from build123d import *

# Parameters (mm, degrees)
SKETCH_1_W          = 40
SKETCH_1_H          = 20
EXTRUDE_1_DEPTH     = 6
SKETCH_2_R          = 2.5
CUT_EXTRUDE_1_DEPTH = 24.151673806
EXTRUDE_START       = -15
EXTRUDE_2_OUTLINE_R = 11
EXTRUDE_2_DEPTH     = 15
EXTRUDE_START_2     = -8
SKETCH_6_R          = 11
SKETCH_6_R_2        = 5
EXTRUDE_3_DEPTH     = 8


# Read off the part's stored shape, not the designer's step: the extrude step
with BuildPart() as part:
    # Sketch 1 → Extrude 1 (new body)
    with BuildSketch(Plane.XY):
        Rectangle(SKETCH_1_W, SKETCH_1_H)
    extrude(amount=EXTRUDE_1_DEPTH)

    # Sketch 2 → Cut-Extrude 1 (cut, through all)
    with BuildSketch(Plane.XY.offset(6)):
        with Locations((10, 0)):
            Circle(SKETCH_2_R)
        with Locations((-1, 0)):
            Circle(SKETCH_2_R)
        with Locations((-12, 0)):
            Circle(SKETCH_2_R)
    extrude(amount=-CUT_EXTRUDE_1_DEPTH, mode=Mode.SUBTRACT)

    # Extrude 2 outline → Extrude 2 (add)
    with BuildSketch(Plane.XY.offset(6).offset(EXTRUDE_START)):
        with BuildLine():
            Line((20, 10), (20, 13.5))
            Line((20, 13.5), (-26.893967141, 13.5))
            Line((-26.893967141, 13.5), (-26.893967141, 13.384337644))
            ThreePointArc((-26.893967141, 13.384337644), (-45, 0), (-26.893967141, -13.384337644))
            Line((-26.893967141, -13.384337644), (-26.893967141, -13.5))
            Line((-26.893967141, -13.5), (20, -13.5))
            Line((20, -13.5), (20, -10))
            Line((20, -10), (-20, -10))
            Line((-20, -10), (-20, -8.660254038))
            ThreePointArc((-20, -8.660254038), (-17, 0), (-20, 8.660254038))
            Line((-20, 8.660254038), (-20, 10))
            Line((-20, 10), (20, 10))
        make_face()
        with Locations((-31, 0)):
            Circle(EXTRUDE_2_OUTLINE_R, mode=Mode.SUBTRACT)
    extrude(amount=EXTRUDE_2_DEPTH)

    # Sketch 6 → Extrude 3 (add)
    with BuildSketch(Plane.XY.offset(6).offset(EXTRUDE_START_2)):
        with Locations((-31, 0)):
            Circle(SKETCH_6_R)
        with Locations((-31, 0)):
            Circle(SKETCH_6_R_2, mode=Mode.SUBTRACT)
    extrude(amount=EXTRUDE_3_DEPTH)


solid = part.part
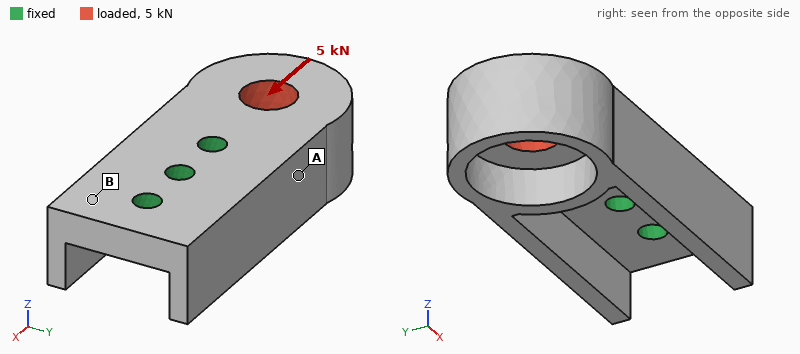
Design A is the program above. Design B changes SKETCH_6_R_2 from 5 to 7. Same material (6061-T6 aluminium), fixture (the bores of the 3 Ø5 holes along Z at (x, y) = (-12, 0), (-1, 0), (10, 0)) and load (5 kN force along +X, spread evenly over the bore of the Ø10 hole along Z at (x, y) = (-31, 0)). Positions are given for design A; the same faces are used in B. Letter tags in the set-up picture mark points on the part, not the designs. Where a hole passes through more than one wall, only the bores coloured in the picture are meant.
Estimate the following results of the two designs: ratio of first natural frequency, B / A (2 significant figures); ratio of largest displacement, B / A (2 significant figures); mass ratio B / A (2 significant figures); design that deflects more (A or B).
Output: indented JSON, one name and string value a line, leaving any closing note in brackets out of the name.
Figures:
{
  "ratio of first natural frequency, B / A": "1.0",
  "ratio of largest displacement, B / A": "1.4",
  "mass ratio B / A": "0.96",
  "design that deflects more": "B"
}
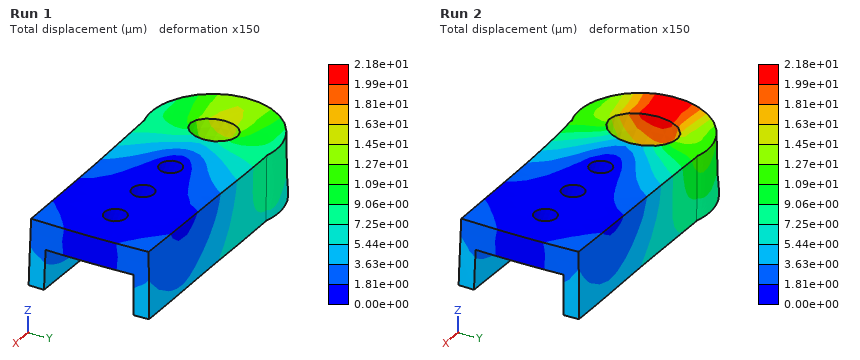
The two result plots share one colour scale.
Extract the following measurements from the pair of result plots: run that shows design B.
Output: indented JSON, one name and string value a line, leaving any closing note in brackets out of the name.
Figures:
{
  "run that shows design B": "Run 2"
}
